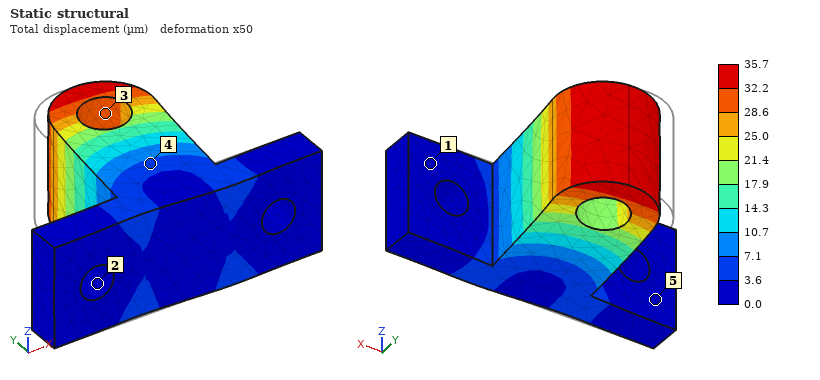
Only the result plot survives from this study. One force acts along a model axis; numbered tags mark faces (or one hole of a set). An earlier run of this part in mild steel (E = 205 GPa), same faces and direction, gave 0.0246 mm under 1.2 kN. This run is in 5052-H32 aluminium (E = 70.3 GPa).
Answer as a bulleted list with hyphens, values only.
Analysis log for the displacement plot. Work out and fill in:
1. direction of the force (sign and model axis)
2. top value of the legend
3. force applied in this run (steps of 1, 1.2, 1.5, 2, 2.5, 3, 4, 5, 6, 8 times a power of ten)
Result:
- +X
- 35.7 µm
- 600 N
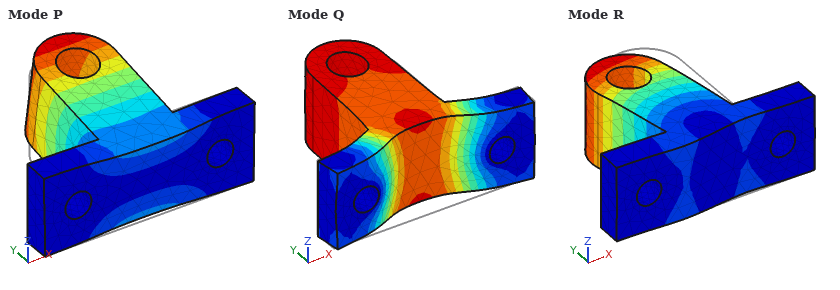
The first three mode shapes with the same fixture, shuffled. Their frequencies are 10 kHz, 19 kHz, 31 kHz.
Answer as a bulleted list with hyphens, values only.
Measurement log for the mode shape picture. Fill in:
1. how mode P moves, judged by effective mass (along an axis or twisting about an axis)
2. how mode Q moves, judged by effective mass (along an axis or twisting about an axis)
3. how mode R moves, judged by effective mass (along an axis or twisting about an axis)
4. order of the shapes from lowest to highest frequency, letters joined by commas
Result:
- along Z
- along Y
- along X
- P, R, Q
